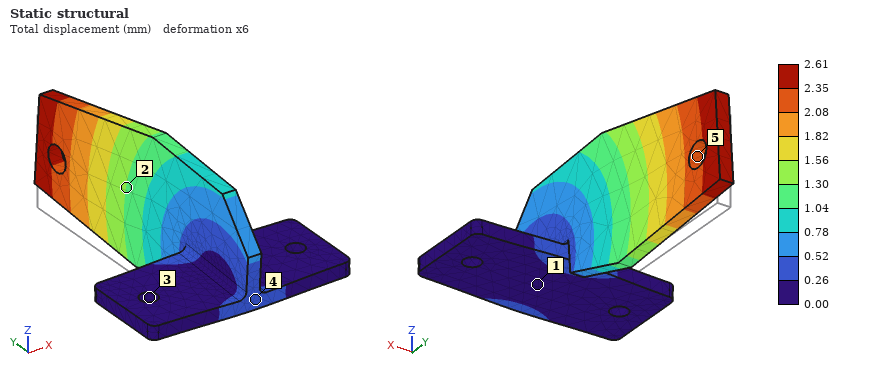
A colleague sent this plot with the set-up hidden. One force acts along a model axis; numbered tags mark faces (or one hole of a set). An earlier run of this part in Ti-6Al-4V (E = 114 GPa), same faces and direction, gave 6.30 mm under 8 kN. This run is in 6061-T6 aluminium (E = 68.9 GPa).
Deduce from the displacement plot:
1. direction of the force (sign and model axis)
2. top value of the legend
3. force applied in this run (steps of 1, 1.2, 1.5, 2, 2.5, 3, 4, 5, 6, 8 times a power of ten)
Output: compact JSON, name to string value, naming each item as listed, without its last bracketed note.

{"direction of the force": "+Z", "top value of the legend": "2.61 mm", "force applied in this run": "2 kN"}
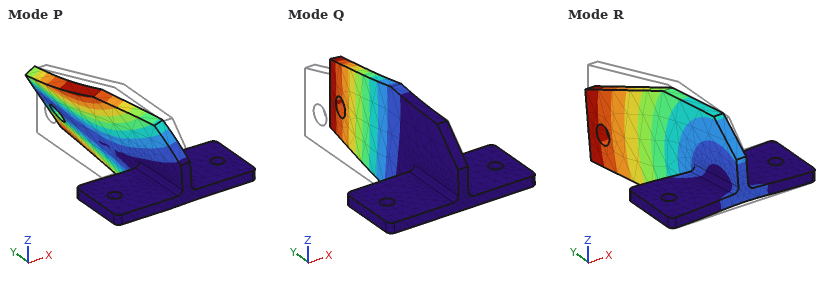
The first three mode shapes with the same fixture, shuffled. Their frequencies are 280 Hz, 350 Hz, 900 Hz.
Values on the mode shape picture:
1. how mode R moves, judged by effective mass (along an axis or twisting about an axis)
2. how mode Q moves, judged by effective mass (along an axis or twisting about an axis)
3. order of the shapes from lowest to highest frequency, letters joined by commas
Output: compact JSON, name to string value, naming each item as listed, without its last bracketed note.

{"how mode R moves, judged by effective mass": "along Z", "how mode Q moves, judged by effective mass": "along X", "order of the shapes from lowest to highest frequency, letters joined by commas": "Q, R, P"}
